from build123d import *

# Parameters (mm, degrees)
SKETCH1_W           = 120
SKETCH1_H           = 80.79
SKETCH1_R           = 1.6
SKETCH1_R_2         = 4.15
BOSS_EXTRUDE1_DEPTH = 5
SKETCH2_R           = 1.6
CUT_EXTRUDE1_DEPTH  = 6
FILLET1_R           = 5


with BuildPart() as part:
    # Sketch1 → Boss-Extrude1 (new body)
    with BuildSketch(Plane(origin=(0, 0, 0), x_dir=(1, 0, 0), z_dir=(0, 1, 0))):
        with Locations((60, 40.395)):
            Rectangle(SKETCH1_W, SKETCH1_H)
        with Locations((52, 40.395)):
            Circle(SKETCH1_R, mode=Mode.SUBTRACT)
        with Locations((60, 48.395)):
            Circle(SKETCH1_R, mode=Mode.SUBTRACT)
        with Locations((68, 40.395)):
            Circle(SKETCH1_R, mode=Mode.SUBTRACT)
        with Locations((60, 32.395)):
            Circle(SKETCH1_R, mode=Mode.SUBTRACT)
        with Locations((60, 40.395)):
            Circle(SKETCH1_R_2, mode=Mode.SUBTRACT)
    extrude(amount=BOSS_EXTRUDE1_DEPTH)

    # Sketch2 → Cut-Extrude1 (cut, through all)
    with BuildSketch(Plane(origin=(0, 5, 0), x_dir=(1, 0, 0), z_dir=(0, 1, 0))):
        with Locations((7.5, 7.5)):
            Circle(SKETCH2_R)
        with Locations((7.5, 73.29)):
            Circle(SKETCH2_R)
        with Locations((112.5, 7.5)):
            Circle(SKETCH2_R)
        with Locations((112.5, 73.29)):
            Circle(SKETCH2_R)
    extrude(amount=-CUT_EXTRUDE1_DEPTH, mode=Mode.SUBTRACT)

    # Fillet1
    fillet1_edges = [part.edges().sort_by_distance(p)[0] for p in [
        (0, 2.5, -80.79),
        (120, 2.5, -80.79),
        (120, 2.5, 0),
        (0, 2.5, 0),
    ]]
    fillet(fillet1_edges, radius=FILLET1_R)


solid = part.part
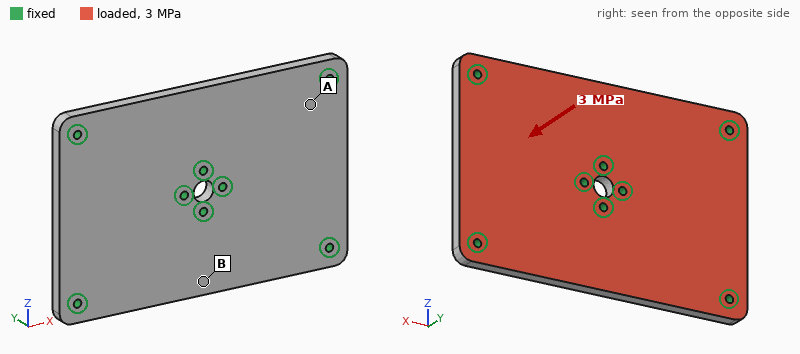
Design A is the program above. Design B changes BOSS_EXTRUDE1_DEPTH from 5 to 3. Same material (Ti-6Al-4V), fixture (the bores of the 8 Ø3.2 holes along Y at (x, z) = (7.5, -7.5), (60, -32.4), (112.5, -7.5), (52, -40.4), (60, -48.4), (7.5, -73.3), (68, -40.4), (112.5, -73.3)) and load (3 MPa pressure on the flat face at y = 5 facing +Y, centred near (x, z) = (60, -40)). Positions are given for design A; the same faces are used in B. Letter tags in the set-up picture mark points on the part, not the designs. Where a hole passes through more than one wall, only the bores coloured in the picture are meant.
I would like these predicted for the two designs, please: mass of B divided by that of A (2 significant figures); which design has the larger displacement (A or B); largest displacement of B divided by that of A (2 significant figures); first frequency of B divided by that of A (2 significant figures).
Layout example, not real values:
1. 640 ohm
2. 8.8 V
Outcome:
1. 0.60
2. B
3. 4.2
4. 0.64
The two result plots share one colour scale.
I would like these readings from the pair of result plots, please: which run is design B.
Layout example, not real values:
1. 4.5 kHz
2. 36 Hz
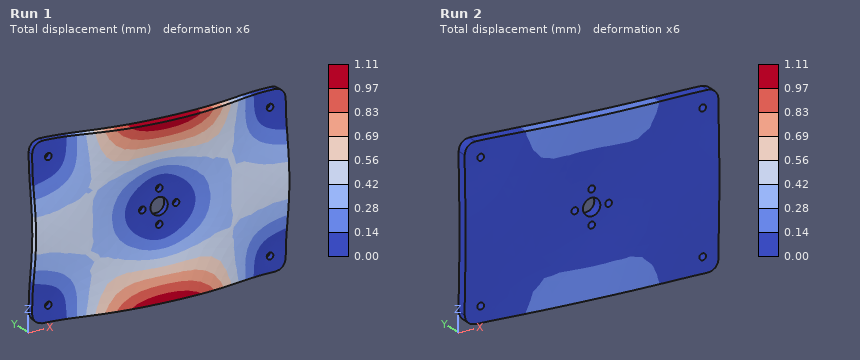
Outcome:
1. Run 1
